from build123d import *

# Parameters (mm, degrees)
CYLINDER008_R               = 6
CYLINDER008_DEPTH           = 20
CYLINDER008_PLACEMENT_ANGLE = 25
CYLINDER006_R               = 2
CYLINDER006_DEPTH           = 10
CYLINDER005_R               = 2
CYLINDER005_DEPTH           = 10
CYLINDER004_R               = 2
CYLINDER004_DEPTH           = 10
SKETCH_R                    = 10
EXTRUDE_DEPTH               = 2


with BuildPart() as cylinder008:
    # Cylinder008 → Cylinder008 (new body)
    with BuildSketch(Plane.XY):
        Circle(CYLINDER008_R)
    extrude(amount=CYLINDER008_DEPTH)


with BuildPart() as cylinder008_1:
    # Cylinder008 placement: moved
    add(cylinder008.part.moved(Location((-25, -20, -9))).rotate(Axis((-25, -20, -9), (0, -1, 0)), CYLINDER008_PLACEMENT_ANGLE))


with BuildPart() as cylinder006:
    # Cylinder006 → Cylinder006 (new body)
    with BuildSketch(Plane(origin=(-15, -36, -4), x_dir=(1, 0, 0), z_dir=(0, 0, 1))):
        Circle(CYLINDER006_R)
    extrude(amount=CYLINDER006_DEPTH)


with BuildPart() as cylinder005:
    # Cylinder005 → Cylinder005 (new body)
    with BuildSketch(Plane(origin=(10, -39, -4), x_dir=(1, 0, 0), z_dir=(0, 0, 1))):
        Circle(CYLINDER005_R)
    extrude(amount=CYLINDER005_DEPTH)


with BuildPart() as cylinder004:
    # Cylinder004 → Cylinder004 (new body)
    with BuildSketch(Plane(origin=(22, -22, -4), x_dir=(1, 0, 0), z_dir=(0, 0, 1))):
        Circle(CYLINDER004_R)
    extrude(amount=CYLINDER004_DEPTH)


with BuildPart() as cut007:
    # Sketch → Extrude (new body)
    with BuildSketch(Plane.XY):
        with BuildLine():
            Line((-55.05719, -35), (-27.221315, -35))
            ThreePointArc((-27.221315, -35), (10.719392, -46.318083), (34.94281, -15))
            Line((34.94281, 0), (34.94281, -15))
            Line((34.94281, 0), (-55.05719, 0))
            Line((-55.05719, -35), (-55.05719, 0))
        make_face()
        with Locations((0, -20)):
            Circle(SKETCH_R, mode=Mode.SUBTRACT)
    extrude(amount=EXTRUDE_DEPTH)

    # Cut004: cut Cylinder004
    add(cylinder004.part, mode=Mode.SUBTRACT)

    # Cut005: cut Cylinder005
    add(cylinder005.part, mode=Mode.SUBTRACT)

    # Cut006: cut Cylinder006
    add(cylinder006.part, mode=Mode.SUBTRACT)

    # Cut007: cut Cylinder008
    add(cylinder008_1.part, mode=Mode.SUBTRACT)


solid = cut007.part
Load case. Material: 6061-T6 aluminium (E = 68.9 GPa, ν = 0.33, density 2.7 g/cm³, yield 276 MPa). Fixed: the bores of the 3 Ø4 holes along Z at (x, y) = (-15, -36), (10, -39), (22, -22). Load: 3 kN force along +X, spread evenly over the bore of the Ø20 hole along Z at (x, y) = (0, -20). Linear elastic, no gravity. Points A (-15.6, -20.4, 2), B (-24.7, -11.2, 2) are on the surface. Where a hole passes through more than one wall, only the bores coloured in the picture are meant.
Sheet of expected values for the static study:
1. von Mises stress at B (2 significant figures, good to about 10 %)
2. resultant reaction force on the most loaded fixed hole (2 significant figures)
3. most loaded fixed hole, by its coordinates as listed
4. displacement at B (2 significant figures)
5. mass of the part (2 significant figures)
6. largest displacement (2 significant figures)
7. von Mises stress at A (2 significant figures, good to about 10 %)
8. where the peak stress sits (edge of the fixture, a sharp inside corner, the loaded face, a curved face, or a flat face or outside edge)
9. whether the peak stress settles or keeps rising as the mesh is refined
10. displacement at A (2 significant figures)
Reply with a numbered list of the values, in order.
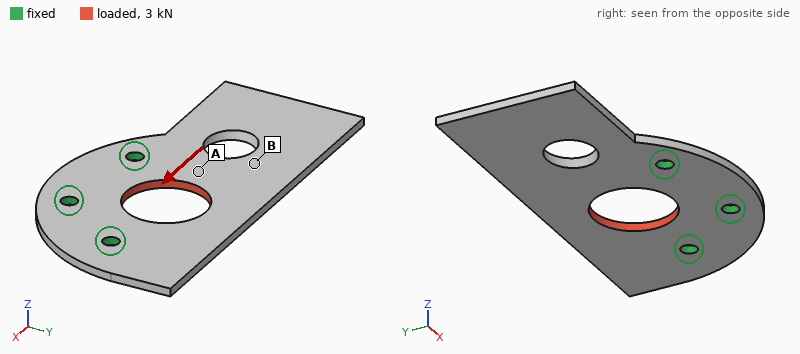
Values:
1. 13 MPa
2. 1.8 kN
3. (22, -22)
4. 33 µm
5. 17 g
6. 59 µm
7. 33 MPa
8. edge of the fixture
9. keeps rising
10. 25 µm
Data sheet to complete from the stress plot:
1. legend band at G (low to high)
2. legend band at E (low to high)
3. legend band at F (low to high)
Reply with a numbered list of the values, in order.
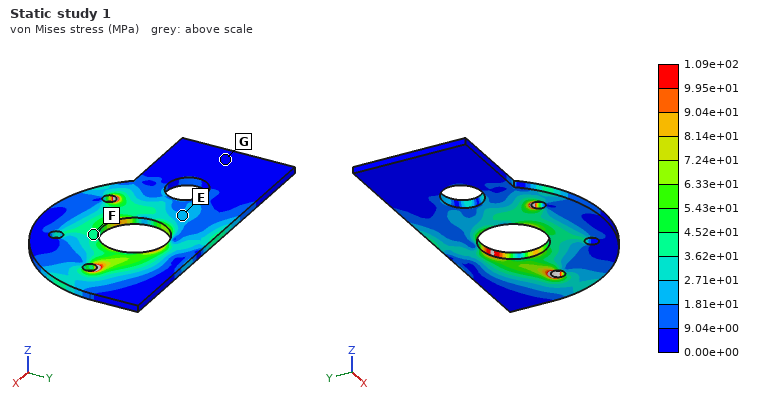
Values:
1. 0.00e+00 to 9.04e+00 MPa
2. 1.81e+01 to 2.71e+01 MPa
3. 3.62e+01 to 4.52e+01 MPa
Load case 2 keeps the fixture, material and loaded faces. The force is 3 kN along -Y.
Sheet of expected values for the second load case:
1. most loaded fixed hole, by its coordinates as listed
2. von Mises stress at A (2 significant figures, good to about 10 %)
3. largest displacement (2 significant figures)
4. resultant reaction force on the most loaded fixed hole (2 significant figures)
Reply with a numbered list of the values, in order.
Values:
1. (-15, -36)
2. 36 MPa
3. 25 µm
4. 1.5 kN
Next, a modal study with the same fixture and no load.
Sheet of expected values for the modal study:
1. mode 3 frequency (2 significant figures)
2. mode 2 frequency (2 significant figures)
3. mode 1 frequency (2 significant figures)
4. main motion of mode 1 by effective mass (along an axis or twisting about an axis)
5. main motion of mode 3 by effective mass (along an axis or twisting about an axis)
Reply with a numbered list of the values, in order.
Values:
1. 2900 Hz
2. 1500 Hz
3. 660 Hz
4. along Z
5. along Z
